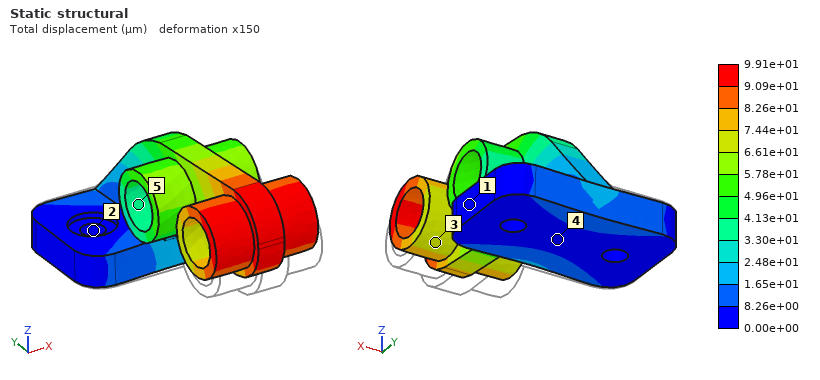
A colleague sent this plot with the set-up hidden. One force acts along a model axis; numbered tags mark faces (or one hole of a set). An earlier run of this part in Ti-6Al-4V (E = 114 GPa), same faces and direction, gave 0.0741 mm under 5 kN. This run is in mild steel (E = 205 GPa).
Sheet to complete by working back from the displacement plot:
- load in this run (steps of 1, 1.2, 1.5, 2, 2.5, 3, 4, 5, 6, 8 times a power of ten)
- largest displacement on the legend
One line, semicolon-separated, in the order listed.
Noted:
12 kN; 9.91e+01 µm
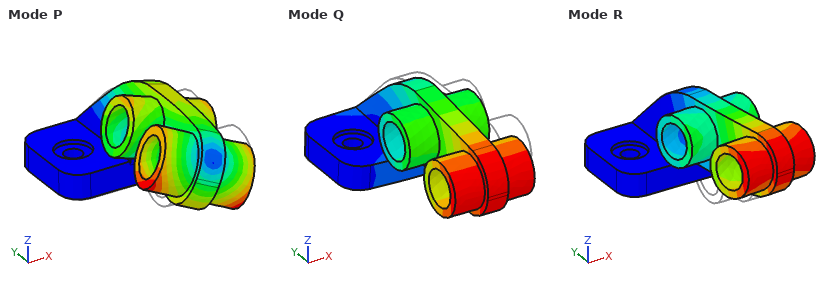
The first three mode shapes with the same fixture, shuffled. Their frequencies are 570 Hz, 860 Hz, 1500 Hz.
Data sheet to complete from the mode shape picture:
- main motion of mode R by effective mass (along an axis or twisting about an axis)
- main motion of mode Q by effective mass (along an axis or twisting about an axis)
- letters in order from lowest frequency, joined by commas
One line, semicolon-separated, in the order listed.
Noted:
along X; along Z; R, Q, P
